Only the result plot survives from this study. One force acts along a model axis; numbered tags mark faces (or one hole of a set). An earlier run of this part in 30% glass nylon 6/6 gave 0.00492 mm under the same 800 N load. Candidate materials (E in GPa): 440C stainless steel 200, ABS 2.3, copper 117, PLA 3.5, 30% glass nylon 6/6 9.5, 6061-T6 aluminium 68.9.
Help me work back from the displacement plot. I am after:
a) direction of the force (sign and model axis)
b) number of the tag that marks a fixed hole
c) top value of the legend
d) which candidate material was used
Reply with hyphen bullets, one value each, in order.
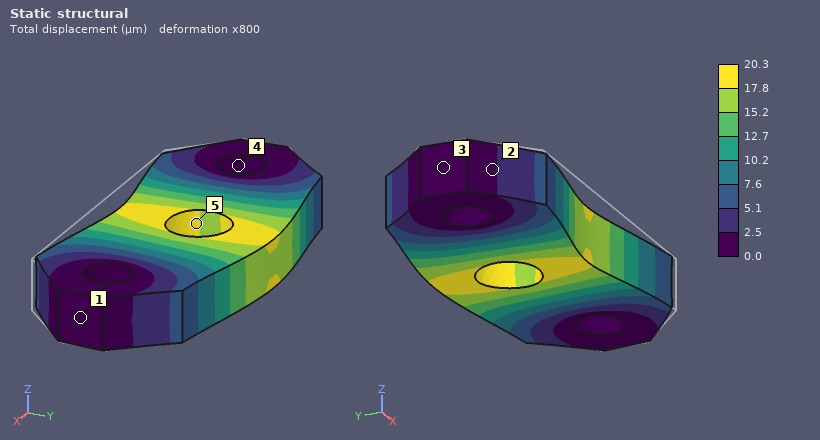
- +Y
- 4
- 20.3 µm
- ABS
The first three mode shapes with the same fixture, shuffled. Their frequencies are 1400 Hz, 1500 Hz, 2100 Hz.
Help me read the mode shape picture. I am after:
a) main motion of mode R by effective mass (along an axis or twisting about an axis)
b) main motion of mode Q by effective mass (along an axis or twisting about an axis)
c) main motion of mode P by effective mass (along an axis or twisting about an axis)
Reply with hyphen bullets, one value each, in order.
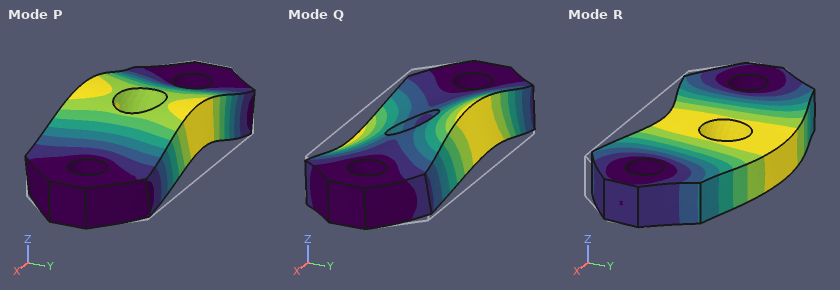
- along Y
- twisting about X
- along Z
